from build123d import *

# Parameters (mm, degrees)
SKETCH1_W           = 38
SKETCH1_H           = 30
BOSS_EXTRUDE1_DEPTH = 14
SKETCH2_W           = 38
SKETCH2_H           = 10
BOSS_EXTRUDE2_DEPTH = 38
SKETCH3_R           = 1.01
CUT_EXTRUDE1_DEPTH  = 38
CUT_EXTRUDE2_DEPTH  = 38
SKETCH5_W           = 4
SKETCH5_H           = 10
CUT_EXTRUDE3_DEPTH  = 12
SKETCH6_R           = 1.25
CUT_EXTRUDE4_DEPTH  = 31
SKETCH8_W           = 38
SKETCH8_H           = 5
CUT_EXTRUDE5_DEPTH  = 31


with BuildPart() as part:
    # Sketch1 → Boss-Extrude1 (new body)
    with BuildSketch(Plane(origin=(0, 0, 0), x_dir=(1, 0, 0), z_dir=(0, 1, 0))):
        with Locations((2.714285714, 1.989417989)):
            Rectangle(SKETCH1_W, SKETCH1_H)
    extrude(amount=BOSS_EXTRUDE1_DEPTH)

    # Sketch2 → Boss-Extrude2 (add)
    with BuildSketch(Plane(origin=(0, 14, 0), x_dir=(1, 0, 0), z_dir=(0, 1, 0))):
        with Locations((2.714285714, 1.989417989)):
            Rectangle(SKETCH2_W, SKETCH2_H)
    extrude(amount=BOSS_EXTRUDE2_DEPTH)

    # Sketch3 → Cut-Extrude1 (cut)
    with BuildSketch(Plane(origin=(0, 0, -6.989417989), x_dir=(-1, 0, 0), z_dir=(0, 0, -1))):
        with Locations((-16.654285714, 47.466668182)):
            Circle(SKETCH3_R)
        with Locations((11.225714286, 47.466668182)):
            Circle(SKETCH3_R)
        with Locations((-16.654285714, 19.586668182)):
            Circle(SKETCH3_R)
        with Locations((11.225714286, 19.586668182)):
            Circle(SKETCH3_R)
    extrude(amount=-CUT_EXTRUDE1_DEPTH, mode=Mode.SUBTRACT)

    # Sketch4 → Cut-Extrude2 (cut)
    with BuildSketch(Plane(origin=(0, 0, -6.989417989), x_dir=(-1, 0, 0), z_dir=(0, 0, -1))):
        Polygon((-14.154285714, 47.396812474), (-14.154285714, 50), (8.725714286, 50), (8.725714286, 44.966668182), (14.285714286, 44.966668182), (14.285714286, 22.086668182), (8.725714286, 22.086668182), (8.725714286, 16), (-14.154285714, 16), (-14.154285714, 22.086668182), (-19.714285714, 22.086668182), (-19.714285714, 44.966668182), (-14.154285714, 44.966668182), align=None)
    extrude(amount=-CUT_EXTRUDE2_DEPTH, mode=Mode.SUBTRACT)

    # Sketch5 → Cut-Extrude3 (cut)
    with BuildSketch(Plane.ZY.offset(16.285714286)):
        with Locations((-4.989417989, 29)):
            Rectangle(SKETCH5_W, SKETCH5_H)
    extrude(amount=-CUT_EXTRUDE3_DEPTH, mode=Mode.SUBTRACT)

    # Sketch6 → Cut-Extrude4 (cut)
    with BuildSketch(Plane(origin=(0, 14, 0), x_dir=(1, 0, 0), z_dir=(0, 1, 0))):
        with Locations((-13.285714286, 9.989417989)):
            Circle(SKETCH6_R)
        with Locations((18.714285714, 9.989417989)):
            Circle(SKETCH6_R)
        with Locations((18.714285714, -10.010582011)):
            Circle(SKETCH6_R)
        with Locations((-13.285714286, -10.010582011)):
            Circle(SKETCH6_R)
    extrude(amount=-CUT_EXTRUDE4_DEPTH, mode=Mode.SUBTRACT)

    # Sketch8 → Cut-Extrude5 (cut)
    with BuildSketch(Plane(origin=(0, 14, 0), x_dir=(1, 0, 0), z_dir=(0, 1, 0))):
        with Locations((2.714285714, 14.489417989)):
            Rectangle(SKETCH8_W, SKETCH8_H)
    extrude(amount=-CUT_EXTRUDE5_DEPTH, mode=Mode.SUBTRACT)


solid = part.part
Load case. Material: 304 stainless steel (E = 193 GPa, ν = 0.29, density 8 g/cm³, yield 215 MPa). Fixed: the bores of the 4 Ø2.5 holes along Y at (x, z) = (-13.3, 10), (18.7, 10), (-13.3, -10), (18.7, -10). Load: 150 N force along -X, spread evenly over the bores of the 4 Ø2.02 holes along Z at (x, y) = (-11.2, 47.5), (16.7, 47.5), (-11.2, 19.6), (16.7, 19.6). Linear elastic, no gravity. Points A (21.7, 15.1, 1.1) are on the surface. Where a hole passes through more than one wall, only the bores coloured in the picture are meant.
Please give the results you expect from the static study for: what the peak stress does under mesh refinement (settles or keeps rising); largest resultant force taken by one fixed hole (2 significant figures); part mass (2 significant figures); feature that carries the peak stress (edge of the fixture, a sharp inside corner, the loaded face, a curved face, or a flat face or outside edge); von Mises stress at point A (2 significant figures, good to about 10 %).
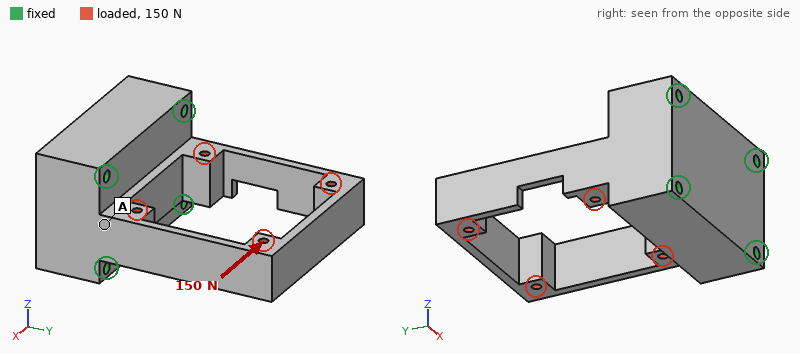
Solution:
keeps rising
79 N
140 g
a sharp inside corner
9.2 MPa
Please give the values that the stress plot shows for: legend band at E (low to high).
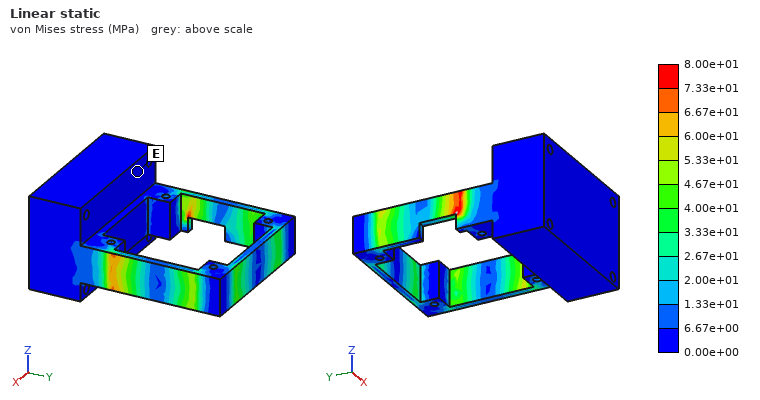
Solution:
0.00e+00 to 6.67e+00 MPa
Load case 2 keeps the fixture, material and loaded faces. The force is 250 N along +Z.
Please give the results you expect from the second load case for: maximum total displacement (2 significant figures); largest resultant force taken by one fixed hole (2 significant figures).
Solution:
63 µm
180 N
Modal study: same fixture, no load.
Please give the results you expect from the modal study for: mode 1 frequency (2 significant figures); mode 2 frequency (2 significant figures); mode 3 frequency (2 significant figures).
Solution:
1500 Hz
2200 Hz
4100 Hz
